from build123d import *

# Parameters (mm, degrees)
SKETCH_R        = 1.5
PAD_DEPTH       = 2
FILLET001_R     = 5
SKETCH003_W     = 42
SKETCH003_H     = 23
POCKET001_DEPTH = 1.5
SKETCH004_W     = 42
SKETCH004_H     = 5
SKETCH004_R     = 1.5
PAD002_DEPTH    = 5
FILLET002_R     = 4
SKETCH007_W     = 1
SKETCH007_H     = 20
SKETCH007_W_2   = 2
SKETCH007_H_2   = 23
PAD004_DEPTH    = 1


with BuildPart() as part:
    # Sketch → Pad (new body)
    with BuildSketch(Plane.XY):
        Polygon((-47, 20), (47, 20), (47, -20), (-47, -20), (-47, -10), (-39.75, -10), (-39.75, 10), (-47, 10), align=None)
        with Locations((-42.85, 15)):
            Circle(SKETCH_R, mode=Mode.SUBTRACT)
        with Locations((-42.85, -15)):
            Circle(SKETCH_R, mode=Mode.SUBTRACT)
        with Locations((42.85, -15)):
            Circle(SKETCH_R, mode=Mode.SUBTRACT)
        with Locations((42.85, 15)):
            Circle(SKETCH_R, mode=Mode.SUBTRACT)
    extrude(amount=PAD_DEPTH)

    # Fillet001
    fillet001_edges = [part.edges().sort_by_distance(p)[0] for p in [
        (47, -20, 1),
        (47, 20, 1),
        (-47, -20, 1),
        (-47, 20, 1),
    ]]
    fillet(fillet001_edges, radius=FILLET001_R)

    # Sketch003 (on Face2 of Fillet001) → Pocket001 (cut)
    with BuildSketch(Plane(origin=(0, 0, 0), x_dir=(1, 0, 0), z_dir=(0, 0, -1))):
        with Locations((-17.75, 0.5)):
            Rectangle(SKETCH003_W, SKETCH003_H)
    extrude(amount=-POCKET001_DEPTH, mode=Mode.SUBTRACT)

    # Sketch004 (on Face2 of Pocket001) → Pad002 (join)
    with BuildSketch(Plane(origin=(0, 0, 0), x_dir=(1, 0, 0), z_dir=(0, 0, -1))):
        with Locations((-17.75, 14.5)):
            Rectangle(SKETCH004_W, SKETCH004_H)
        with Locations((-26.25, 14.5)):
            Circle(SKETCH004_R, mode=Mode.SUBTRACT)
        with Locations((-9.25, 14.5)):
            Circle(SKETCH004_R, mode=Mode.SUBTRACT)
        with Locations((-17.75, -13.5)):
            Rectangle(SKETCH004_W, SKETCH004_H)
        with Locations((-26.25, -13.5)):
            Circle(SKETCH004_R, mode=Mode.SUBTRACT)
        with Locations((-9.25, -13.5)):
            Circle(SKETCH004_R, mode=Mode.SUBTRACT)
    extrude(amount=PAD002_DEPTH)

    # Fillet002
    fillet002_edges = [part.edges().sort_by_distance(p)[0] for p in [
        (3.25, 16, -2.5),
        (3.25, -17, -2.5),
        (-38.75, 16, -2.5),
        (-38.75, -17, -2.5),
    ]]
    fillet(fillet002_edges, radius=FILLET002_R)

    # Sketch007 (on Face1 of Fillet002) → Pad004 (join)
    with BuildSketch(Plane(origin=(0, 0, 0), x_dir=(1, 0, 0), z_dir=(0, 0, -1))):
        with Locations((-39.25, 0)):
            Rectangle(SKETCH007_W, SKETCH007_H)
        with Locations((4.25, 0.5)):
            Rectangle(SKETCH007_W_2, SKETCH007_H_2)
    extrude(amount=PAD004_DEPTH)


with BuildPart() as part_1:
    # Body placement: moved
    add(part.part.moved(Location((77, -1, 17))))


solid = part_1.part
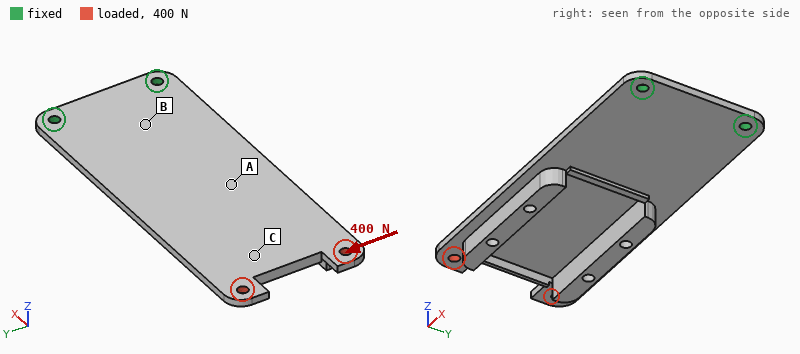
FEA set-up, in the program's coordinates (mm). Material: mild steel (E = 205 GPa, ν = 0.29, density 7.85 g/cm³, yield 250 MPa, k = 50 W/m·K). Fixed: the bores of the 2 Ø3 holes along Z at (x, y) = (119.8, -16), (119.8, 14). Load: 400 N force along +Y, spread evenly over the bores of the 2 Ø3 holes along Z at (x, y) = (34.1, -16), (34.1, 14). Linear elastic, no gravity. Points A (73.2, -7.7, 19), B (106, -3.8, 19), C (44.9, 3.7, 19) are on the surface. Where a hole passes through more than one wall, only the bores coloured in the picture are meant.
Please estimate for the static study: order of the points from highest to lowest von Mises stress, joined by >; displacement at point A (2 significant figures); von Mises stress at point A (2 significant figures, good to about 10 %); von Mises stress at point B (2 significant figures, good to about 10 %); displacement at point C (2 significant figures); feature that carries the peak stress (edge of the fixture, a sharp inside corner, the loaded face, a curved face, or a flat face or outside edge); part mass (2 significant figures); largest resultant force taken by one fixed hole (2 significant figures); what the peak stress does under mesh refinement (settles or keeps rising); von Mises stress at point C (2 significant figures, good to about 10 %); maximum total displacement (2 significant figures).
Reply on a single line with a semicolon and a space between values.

C > A > B; 21 µm; 39 MPa; 13 MPa; 49 µm; a sharp inside corner; 60 g; 1.1 kN; keeps rising; 53 MPa; 88 µm
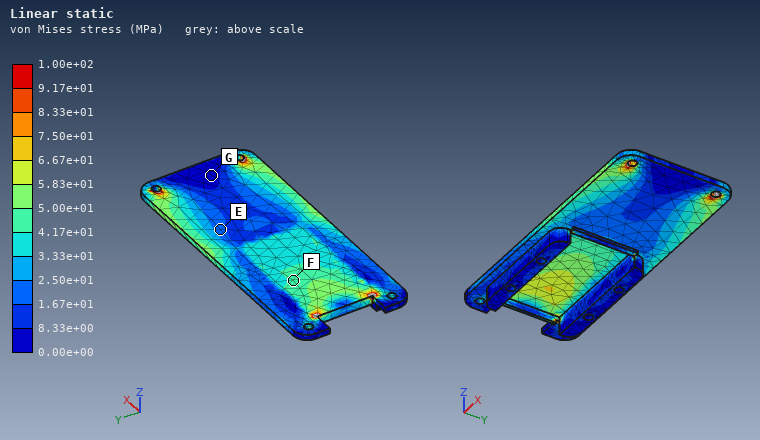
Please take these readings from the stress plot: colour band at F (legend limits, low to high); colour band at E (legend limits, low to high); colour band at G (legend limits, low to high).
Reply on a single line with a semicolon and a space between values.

4.17e+01 to 5.00e+01 MPa; 1.67e+01 to 2.50e+01 MPa; 0.00e+00 to 8.33e+00 MPa
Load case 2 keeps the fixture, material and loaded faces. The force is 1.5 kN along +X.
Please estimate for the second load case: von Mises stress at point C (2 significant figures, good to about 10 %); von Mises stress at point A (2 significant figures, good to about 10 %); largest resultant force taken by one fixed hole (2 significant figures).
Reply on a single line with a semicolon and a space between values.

19 MPa; 36 MPa; 760 N
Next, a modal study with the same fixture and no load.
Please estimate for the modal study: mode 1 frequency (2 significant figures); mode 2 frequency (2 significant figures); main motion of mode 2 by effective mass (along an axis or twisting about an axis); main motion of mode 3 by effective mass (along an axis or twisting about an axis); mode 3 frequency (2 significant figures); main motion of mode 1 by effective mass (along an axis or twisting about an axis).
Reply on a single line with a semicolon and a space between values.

210 Hz; 820 Hz; twisting about X; along Z; 1600 Hz; along Z
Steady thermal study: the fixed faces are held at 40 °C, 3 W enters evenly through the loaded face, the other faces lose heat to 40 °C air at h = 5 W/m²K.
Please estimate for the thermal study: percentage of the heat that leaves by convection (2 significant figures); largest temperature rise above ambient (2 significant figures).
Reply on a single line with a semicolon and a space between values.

38 %; 58 K
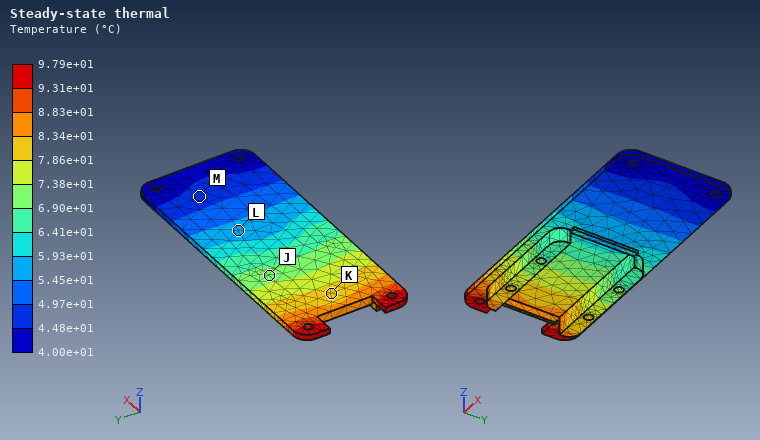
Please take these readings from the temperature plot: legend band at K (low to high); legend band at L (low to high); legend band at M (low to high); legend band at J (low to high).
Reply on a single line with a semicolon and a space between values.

7.86e+01 to 8.34e+01 °C; 5.45e+01 to 5.93e+01 °C; 4.48e+01 to 4.97e+01 °C; 6.90e+01 to 7.38e+01 °C
